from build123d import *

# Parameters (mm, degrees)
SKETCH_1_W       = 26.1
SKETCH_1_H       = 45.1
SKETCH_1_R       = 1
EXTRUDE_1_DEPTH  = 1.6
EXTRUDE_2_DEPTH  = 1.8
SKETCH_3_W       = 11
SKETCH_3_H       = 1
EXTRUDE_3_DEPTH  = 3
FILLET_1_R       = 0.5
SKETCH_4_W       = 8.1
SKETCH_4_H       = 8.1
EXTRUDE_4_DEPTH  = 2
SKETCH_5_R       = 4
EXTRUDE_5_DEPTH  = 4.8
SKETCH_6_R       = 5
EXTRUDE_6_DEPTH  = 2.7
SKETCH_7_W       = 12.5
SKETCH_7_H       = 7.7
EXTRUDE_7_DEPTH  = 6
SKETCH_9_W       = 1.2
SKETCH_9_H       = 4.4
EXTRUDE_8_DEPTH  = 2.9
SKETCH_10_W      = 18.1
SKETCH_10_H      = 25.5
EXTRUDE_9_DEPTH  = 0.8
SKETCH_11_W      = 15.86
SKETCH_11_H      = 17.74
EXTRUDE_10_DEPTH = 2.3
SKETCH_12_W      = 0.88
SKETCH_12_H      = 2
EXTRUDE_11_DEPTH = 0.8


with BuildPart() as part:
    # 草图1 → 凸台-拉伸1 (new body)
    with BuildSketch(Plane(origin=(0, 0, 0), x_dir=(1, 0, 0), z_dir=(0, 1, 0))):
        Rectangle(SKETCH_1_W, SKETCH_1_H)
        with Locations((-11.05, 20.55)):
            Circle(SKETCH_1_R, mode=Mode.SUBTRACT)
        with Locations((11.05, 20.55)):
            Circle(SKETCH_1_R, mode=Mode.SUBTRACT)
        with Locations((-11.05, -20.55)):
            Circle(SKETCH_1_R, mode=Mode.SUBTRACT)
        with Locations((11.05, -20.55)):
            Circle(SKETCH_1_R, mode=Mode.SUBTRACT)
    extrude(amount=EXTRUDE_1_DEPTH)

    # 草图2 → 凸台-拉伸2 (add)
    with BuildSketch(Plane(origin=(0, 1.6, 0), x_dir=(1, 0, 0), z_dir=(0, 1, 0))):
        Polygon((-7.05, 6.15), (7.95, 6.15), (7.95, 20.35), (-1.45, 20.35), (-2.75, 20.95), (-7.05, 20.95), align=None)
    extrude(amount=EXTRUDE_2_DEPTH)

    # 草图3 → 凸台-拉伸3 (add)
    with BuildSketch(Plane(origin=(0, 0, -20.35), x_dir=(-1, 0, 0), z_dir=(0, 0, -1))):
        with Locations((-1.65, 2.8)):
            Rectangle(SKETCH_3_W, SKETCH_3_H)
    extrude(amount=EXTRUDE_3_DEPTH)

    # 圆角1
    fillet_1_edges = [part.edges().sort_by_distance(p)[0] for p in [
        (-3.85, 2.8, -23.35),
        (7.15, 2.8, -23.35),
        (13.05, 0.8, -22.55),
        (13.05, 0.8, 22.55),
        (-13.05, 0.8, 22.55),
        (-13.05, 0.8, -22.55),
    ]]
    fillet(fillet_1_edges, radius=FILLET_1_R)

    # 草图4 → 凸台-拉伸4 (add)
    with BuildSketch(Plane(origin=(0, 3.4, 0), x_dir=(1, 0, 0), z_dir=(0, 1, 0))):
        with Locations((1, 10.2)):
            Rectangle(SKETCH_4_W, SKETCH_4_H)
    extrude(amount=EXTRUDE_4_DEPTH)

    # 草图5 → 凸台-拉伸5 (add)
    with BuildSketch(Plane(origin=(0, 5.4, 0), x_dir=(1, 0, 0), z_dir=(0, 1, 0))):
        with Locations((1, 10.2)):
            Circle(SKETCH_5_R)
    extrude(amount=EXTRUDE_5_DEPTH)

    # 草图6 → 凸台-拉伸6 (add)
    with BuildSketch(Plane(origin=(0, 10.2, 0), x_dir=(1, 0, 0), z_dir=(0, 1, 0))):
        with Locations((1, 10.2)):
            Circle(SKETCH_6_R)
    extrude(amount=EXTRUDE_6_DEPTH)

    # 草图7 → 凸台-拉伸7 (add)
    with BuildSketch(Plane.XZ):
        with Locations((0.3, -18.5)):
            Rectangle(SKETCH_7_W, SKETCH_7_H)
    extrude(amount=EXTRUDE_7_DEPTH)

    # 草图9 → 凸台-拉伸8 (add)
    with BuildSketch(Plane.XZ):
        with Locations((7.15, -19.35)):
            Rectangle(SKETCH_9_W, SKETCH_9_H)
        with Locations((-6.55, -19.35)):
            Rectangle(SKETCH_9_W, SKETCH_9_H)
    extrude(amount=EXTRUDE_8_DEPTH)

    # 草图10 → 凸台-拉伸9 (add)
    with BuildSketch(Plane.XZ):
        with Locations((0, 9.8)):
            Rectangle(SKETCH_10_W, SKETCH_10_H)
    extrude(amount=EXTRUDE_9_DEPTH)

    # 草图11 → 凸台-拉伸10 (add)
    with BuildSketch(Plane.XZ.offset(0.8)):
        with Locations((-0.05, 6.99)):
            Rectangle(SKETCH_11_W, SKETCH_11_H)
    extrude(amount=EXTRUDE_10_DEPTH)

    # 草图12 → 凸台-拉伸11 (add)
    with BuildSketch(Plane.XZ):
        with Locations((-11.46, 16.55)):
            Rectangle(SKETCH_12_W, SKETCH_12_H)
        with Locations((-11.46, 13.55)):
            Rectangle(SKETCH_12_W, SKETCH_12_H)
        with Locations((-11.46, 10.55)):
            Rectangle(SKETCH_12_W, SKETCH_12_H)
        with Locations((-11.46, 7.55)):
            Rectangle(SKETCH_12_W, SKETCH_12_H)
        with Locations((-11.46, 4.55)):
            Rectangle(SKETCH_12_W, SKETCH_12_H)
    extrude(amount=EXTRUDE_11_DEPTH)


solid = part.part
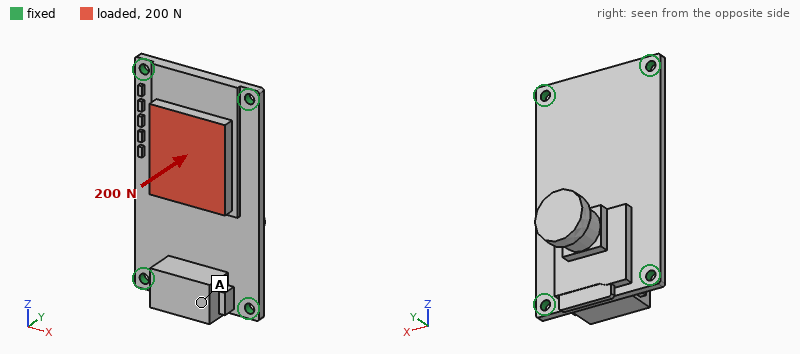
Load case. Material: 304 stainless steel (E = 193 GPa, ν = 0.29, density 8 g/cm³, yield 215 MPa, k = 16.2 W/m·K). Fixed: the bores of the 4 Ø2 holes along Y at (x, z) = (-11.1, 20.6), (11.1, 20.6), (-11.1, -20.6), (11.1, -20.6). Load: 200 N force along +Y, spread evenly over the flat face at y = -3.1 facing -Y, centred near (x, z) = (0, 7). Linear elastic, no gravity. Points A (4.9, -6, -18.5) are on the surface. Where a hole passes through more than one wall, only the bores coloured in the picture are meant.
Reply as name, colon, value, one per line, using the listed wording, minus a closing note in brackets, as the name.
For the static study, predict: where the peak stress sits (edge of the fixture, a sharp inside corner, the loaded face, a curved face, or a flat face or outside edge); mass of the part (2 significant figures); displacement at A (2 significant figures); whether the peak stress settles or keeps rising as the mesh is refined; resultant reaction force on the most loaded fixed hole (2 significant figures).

where the peak stress sits: edge of the fixture
mass of the part: 36 g
displacement at A: 7.3 µm
whether the peak stress settles or keeps rising as the mesh is refined: keeps rising
resultant reaction force on the most loaded fixed hole: 88 N
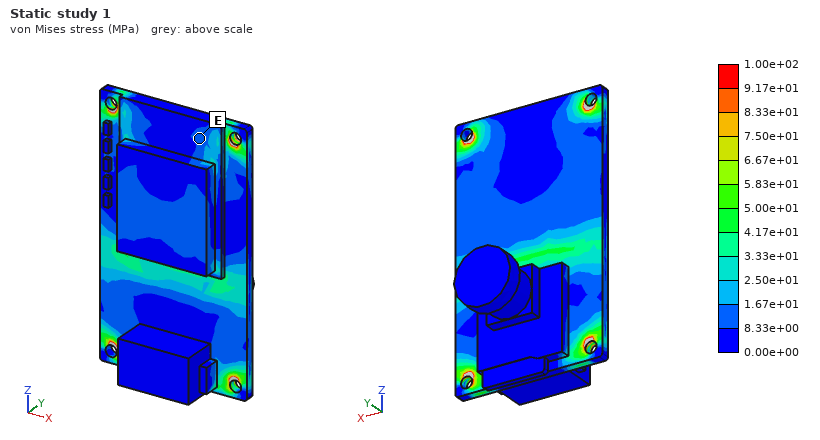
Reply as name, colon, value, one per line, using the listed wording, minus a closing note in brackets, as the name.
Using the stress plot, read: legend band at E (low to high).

legend band at E: 8.33e+00 to 1.67e+01 MPa
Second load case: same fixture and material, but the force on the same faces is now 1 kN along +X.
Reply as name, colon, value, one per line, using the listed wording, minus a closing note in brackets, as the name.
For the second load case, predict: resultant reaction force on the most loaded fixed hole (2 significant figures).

resultant reaction force on the most loaded fixed hole: 510 N
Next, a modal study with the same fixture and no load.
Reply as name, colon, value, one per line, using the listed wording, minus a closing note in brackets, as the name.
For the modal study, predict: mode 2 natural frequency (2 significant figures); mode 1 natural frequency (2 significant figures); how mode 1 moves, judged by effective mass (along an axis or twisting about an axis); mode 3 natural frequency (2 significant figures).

mode 2 natural frequency: 12 kHz
mode 1 natural frequency: 3600 Hz
how mode 1 moves, judged by effective mass: along Y
mode 3 natural frequency: 14 kHz
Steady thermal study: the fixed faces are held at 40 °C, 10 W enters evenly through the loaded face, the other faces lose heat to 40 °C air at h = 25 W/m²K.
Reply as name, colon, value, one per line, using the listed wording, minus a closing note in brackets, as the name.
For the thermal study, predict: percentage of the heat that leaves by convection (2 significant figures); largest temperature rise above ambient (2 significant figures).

percentage of the heat that leaves by convection: 34 %
largest temperature rise above ambient: 86 K
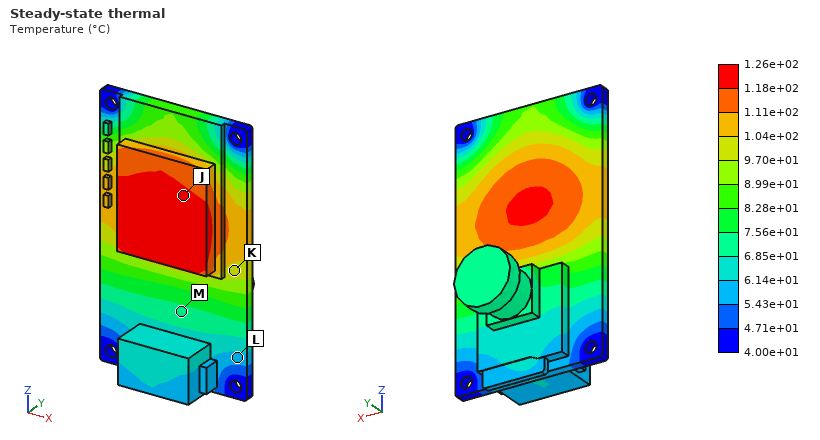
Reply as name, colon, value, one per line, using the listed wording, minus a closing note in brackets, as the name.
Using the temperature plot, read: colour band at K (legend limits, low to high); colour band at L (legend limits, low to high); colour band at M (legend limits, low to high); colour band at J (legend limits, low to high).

colour band at K: 9.70e+01 to 1.04e+02 °C
colour band at L: 5.43e+01 to 6.14e+01 °C
colour band at M: 6.85e+01 to 7.56e+01 °C
colour band at J: 1.18e+02 to 1.26e+02 °C
